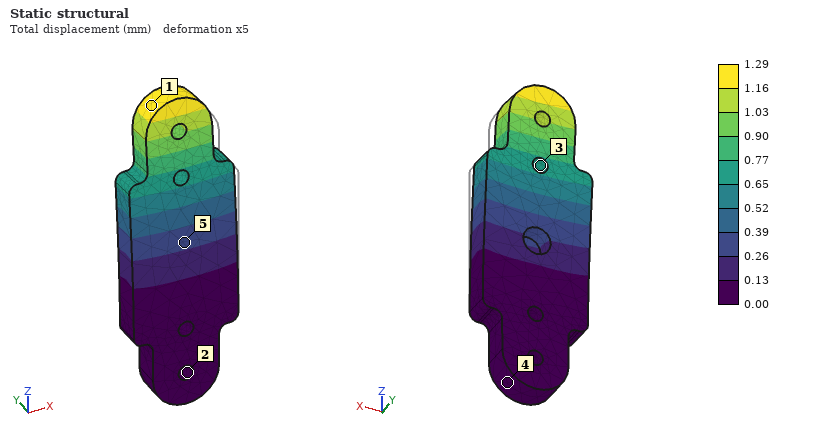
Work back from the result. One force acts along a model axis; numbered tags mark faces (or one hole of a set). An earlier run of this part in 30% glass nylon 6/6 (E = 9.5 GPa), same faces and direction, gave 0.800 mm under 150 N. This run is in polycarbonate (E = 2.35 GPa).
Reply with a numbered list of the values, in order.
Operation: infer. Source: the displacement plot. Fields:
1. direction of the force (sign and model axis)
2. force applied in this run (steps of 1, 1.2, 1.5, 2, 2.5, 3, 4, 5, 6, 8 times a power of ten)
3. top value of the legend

1. +Y
2. 60 N
3. 1.29 mm
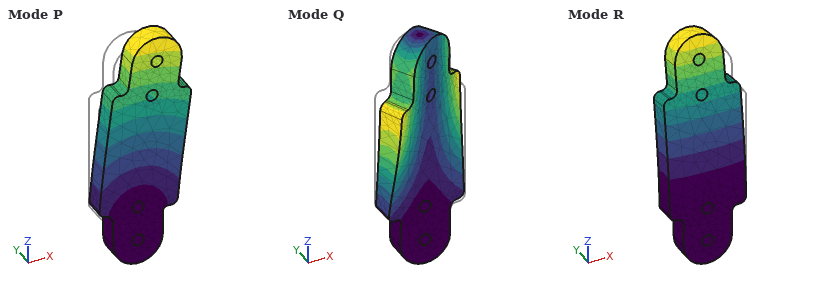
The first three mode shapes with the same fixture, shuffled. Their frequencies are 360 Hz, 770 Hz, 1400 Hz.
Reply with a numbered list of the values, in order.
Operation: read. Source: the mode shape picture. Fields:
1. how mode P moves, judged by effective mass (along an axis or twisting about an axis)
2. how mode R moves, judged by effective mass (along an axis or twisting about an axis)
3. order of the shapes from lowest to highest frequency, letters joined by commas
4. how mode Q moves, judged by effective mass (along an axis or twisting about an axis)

1. along X
2. along Y
3. R, P, Q
4. twisting about Z
